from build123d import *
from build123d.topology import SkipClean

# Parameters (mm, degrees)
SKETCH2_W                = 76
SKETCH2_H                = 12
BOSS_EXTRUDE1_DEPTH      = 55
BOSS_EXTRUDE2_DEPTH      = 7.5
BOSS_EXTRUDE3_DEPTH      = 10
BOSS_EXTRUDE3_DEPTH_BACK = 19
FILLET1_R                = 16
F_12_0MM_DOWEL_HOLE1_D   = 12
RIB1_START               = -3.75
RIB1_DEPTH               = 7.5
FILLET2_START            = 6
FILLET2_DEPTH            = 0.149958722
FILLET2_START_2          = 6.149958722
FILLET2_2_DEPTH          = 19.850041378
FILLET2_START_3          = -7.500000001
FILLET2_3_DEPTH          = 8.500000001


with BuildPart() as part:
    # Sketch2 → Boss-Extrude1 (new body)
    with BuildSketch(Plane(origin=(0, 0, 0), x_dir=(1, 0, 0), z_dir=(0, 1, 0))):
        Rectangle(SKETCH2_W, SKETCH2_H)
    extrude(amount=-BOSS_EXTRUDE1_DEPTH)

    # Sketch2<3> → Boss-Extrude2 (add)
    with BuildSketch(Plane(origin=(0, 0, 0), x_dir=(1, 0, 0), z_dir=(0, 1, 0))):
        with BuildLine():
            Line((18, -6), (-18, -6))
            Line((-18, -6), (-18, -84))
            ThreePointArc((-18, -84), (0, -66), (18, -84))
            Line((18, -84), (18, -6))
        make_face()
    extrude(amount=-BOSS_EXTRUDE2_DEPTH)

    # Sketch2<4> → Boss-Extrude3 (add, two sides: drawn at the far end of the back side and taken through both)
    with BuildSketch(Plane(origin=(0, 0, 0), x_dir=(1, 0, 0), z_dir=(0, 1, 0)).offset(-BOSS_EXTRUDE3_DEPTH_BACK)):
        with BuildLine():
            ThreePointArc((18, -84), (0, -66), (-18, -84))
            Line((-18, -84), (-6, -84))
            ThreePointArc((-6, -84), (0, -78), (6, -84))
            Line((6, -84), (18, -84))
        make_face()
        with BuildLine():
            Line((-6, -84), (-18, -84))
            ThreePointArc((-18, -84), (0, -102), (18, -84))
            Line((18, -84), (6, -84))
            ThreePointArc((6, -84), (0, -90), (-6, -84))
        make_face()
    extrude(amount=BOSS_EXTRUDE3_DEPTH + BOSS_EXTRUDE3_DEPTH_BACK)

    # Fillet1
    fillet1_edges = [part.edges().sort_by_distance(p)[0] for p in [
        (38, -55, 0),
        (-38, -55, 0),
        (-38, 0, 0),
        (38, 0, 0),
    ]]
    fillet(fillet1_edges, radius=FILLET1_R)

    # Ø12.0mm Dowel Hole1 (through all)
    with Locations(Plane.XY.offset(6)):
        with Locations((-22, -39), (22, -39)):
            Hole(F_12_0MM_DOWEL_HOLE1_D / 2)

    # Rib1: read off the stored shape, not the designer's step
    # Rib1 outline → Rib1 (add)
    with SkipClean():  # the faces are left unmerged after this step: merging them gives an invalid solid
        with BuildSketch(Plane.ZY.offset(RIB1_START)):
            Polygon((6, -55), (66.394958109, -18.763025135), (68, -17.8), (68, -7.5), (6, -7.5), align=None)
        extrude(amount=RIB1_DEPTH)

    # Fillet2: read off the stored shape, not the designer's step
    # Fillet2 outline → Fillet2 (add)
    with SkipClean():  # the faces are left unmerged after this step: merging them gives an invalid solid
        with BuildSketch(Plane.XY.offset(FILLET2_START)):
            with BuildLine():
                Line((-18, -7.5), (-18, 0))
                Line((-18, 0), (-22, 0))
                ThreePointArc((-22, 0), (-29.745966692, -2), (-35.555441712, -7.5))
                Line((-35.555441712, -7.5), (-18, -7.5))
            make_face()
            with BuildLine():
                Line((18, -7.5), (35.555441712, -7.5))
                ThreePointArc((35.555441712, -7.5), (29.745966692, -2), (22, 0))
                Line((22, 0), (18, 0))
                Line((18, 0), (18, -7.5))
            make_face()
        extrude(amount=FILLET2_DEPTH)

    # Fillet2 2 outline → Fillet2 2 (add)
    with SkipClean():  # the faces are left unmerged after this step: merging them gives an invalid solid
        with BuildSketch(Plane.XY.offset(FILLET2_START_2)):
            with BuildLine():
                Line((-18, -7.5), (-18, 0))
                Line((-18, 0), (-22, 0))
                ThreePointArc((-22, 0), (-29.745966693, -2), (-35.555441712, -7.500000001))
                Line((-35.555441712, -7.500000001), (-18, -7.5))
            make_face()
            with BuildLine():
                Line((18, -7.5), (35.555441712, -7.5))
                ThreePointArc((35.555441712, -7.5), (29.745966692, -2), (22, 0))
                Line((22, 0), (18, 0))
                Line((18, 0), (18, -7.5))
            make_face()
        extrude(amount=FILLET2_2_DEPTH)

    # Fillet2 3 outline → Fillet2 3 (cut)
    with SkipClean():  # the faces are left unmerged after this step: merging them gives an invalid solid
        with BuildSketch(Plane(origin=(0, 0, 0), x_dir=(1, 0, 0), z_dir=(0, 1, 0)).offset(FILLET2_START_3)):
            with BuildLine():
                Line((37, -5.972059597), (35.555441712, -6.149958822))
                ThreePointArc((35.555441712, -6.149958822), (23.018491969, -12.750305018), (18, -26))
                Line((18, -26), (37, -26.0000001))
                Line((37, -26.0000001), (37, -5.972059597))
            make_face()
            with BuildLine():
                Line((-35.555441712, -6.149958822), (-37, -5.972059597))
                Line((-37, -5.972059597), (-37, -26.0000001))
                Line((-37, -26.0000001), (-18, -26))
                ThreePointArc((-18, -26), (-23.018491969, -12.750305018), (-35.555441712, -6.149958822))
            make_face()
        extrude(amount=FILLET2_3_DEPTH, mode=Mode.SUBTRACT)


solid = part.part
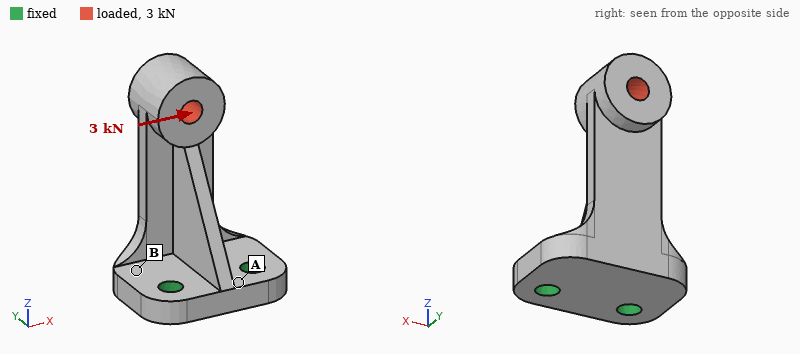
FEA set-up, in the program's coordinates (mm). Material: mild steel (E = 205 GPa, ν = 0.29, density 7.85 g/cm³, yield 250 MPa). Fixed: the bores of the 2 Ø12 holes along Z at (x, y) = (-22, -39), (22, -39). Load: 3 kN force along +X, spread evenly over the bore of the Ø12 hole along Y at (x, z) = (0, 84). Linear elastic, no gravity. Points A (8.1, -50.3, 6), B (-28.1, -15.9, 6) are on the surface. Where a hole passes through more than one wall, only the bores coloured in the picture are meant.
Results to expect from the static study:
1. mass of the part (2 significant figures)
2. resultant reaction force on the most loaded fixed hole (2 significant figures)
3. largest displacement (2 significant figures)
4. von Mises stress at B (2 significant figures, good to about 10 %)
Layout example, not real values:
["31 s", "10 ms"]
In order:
["810 g", "5.8 kN", "0.22 mm", "45 MPa"]
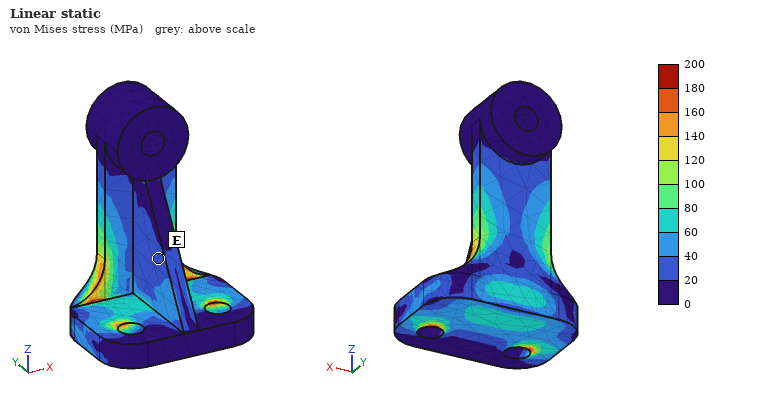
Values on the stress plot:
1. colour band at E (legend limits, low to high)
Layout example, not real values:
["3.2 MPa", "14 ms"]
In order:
["20 to 40 MPa"]
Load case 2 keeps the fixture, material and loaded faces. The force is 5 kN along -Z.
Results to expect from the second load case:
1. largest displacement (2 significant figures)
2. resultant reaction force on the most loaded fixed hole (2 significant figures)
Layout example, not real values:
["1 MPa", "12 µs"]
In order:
["86 µm", "2.5 kN"]
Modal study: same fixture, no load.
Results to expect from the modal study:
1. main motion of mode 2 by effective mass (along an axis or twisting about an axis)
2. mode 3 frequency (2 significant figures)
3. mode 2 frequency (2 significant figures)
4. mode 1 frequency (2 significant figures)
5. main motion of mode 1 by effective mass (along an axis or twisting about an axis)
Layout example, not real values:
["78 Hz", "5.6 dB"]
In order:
["along Y", "2900 Hz", "1400 Hz", "1300 Hz", "along X"]
